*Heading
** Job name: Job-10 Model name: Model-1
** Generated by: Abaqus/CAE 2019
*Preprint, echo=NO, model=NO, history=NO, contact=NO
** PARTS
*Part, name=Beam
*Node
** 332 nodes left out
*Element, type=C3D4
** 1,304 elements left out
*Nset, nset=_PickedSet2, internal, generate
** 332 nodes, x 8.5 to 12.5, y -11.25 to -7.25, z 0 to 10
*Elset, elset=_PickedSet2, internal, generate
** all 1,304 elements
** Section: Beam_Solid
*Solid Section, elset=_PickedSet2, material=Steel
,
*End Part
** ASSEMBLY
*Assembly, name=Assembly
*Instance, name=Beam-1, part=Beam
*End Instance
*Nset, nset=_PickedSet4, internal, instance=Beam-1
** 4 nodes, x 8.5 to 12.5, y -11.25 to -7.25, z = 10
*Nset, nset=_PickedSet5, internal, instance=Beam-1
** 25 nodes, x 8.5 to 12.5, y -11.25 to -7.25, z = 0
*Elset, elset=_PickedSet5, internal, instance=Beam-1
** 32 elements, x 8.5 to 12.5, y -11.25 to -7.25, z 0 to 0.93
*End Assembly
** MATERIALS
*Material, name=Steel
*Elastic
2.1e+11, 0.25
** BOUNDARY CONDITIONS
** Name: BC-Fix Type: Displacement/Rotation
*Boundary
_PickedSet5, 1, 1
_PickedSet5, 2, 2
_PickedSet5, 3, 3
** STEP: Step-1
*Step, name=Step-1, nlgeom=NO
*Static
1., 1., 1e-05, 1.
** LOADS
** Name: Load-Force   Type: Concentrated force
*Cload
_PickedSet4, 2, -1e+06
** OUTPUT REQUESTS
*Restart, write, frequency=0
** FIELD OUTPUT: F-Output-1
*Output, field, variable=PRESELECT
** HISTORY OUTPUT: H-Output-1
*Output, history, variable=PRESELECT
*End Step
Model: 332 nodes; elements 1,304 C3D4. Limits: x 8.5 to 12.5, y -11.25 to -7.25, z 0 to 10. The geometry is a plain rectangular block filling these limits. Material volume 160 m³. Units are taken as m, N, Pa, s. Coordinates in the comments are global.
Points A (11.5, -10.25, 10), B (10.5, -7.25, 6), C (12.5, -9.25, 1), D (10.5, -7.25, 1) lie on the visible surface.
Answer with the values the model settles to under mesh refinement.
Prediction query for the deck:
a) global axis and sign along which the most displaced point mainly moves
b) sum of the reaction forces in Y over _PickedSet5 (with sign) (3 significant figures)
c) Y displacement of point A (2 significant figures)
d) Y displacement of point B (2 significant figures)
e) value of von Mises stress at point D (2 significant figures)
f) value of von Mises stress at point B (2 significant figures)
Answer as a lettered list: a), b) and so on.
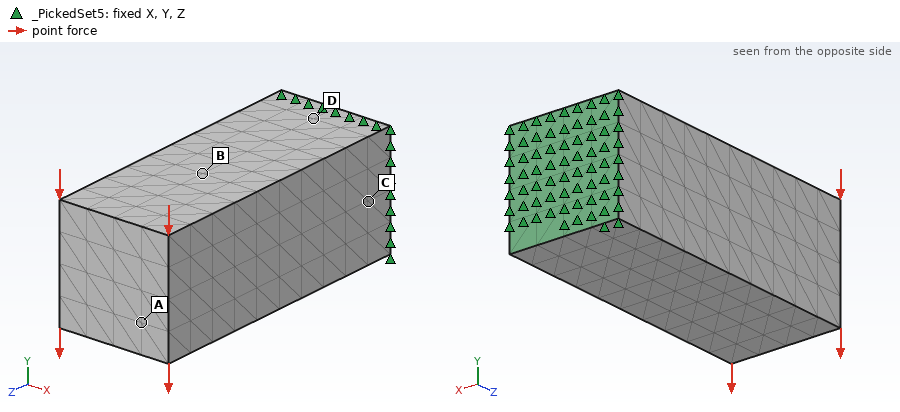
a) -Y
b) 4.00e+06 N
c) -3.3e-04 m
d) -1.5e-04 m
e) 3.2e+06 Pa
f) 1.5e+06 Pa
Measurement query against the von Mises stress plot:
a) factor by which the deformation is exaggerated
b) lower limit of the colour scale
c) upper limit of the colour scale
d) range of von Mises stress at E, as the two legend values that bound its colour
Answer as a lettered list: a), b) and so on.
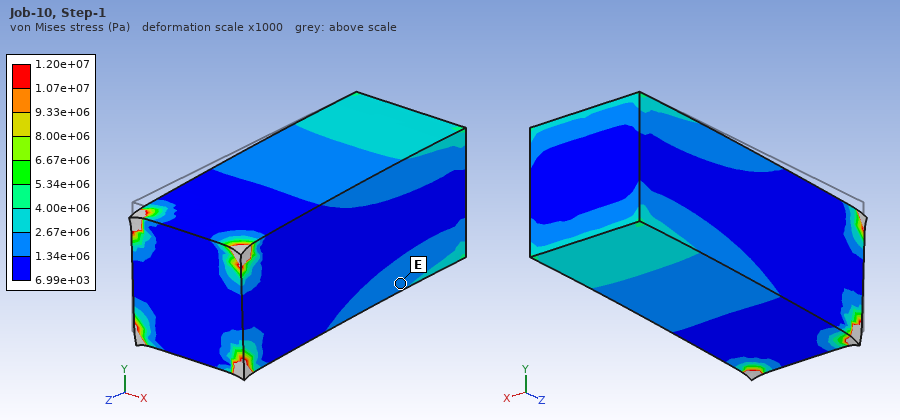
a) 1000
b) 6.99e+03 Pa
c) 1.20e+07 Pa
d) 1.34e+06 to 2.67e+06 Pa
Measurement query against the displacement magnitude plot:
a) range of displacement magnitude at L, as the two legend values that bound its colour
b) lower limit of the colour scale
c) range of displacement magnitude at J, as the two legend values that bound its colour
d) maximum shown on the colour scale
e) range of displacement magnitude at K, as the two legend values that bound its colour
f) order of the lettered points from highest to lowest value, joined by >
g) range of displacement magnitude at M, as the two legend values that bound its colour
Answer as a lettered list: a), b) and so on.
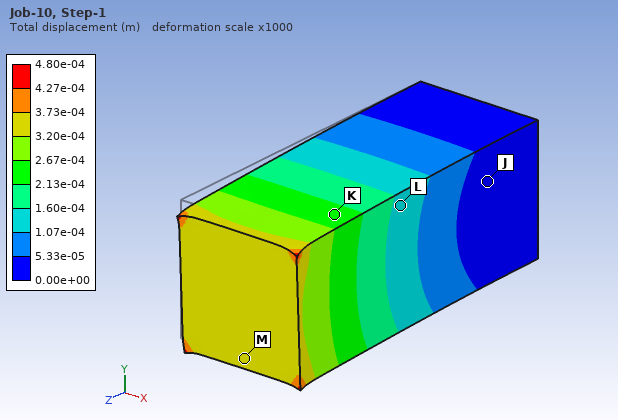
a) 1.07e-04 to 1.60e-04 m
b) 0.00e+00 m
c) 0.00e+00 to 5.33e-05 m
d) 4.80e-04 m
e) 2.13e-04 to 2.67e-04 m
f) M > K > L > J
g) 3.20e-04 to 3.73e-04 m
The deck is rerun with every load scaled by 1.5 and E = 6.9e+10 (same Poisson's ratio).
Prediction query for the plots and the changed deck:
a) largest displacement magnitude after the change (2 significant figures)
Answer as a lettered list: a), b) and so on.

a) 0.0022 m
